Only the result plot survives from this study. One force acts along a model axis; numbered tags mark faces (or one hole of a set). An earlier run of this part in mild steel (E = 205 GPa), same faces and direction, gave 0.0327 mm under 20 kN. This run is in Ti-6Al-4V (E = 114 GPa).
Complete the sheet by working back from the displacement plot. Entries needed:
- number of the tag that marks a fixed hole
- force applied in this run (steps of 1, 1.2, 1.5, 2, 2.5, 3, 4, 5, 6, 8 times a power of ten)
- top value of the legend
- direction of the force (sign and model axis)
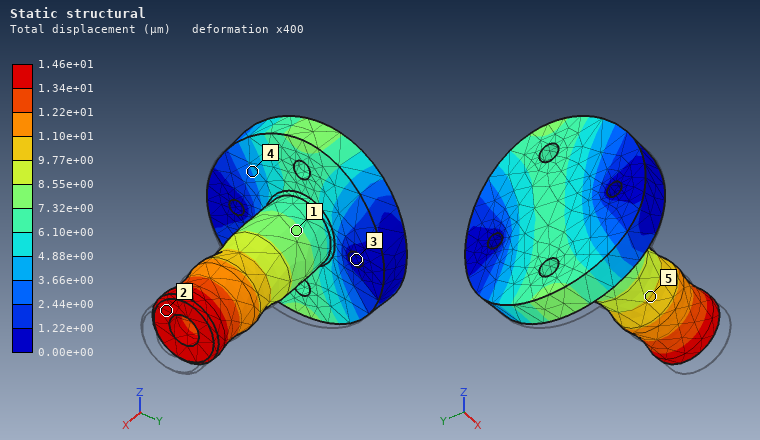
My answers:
3
5 kN
1.46e+01 µm
-X
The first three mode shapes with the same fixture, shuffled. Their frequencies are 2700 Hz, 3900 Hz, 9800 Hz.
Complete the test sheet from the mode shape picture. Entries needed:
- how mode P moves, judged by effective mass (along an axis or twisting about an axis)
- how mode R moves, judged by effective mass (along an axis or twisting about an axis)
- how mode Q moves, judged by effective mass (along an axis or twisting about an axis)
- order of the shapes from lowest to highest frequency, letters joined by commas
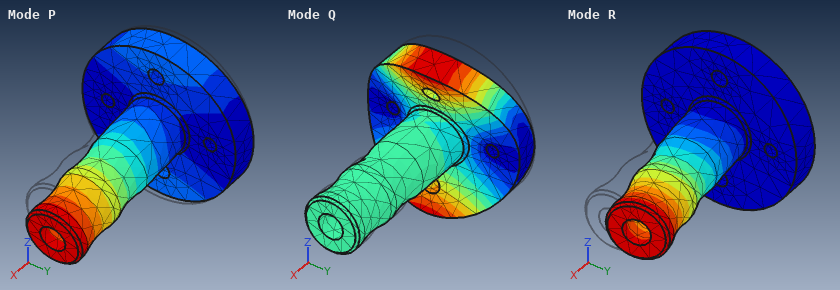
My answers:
along Z
along Y
along X
P, R, Q
